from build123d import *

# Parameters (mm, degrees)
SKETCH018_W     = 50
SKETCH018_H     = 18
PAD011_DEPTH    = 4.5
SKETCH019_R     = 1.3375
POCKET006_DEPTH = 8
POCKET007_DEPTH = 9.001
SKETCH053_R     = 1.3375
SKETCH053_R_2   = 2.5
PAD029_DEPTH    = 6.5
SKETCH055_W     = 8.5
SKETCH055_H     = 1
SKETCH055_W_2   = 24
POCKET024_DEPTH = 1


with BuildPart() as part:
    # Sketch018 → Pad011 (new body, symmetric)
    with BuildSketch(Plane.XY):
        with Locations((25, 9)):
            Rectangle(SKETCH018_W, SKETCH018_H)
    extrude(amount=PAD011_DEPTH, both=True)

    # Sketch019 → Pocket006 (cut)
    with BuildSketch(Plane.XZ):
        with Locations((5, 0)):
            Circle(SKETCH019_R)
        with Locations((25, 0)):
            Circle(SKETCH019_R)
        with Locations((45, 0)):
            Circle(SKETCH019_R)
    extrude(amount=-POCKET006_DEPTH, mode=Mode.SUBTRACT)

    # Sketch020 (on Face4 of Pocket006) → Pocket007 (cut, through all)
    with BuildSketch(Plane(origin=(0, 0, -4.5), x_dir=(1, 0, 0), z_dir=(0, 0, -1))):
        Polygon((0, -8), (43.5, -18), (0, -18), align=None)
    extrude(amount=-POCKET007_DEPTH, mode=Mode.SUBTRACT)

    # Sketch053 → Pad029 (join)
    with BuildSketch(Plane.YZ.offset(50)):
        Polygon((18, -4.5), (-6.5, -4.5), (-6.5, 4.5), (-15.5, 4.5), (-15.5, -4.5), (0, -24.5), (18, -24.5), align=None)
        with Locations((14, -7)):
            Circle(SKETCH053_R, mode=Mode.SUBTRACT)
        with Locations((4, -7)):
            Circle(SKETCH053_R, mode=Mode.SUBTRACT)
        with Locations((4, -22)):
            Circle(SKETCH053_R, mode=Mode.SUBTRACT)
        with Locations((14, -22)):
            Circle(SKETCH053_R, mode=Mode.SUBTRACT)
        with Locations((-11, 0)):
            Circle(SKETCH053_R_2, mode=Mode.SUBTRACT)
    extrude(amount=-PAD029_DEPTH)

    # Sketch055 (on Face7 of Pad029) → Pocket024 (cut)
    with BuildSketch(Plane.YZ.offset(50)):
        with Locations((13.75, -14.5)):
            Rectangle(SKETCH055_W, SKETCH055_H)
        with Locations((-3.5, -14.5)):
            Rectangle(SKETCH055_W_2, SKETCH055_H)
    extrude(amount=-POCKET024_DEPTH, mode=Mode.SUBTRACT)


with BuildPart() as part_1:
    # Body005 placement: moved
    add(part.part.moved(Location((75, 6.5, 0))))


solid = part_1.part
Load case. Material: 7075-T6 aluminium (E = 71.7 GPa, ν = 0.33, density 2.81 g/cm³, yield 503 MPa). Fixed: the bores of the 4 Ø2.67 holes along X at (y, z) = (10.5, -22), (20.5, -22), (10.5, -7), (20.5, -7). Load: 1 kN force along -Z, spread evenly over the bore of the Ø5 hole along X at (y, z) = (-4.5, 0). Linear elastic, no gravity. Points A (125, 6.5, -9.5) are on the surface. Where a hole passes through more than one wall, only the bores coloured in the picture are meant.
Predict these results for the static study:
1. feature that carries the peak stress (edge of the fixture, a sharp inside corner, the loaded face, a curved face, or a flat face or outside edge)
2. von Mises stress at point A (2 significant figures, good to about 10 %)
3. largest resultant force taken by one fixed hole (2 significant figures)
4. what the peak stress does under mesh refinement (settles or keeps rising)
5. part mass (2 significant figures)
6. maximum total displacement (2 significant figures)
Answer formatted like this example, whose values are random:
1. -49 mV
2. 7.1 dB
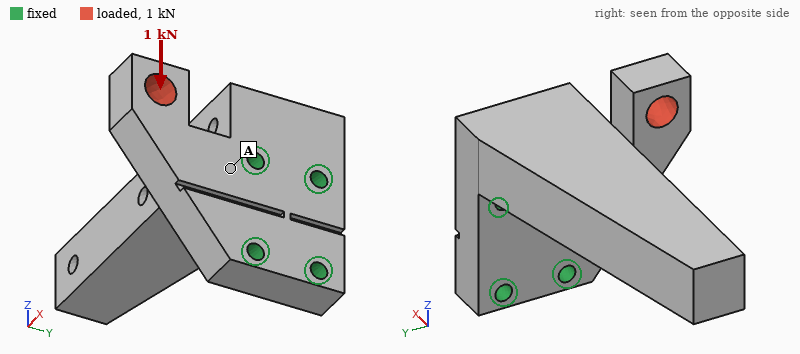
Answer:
1. a sharp inside corner
2. 8.3 MPa
3. 970 N
4. keeps rising
5. 27 g
6. 37 µm
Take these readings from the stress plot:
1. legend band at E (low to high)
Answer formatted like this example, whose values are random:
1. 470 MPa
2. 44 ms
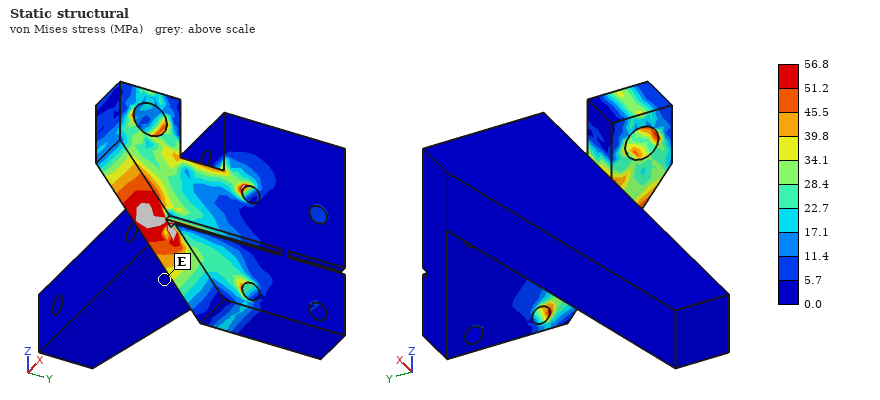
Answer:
1. 0.0 to 5.7 MPa
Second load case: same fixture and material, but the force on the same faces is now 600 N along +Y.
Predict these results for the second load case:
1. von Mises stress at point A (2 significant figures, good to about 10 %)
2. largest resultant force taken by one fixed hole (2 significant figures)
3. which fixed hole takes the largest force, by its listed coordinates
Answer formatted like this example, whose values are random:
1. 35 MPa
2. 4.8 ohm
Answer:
1. 11 MPa
2. 770 N
3. (10.5, -7)
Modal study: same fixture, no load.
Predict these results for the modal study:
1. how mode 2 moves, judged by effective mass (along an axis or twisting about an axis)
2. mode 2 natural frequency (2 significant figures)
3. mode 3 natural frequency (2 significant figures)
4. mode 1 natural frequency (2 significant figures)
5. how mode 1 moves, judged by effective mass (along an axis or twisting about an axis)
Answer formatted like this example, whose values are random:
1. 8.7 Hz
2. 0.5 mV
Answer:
1. along Y
2. 5100 Hz
3. 11 kHz
4. 2900 Hz
5. along Z
